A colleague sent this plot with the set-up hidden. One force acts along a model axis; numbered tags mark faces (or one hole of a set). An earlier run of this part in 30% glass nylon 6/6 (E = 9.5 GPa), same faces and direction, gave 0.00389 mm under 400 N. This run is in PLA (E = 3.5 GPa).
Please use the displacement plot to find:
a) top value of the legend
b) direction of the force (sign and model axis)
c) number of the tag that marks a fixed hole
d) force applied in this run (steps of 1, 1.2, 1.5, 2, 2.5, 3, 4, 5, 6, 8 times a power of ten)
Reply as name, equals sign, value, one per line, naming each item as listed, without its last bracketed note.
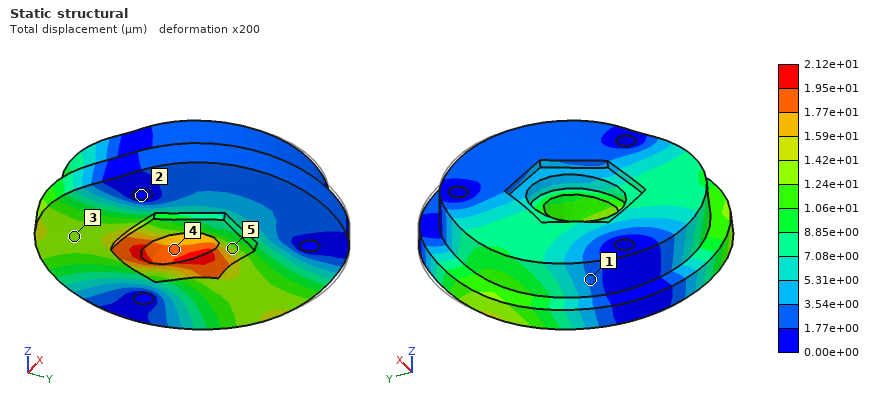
top value of the legend = 2.12e+01 µm
direction of the force = -Y
number of the tag that marks a fixed hole = 2
force applied in this run = 800 N
